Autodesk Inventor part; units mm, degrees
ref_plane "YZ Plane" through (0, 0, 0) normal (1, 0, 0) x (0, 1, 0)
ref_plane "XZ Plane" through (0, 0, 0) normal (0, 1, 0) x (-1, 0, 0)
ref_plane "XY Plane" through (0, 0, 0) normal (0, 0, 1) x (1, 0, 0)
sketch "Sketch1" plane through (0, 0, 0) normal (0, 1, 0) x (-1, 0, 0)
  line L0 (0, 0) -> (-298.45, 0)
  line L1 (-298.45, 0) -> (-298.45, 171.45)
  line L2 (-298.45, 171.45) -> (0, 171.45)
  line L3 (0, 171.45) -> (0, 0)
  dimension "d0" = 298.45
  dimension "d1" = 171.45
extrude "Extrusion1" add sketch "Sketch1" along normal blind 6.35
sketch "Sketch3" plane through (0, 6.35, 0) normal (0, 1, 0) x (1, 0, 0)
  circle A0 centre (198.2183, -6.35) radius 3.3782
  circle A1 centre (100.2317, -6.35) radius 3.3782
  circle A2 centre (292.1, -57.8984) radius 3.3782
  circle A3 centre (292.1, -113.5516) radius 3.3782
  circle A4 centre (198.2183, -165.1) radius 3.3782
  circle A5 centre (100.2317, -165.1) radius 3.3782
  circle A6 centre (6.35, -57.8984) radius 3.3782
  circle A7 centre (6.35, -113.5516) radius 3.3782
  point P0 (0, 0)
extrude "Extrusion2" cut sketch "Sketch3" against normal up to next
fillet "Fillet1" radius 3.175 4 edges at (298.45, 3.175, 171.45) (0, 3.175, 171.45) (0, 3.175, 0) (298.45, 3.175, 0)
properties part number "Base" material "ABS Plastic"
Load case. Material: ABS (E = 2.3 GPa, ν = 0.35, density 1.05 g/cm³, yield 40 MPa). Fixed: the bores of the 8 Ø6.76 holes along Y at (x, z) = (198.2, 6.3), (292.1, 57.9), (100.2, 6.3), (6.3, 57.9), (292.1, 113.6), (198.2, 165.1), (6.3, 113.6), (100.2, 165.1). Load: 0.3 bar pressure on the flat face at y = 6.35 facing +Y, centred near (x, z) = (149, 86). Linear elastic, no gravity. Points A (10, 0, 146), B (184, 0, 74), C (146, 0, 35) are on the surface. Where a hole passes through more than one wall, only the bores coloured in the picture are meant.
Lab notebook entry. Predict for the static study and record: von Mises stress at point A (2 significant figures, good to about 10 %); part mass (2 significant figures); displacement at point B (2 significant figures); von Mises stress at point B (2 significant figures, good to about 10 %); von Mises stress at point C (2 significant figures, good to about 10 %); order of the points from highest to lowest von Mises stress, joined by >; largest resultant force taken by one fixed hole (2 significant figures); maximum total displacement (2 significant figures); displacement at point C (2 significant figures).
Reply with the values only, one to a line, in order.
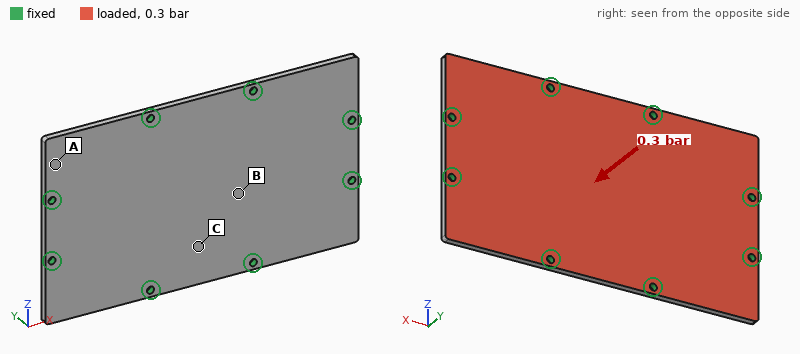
1.2 MPa
340 g
1.2 mm
4.3 MPa
2.4 MPa
B > C > A
240 N
1.3 mm
0.72 mm
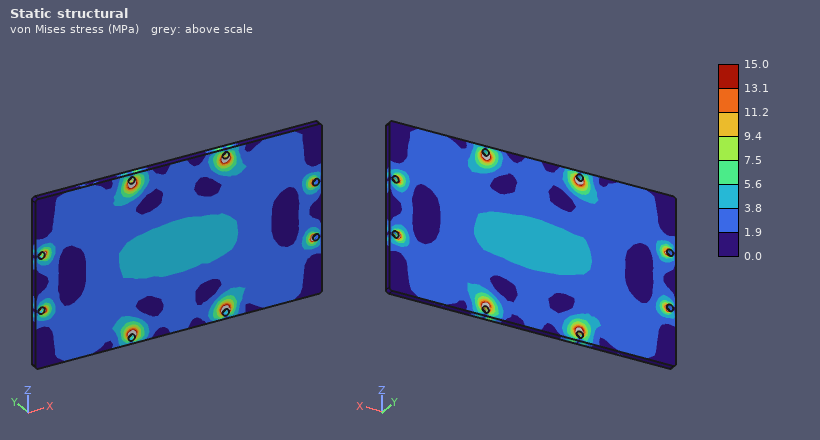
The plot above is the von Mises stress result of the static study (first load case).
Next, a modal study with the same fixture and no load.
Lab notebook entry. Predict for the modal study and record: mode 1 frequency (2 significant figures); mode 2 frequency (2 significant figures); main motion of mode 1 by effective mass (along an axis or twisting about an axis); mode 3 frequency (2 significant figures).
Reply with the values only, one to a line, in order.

350 Hz
530 Hz
along Y
550 Hz
